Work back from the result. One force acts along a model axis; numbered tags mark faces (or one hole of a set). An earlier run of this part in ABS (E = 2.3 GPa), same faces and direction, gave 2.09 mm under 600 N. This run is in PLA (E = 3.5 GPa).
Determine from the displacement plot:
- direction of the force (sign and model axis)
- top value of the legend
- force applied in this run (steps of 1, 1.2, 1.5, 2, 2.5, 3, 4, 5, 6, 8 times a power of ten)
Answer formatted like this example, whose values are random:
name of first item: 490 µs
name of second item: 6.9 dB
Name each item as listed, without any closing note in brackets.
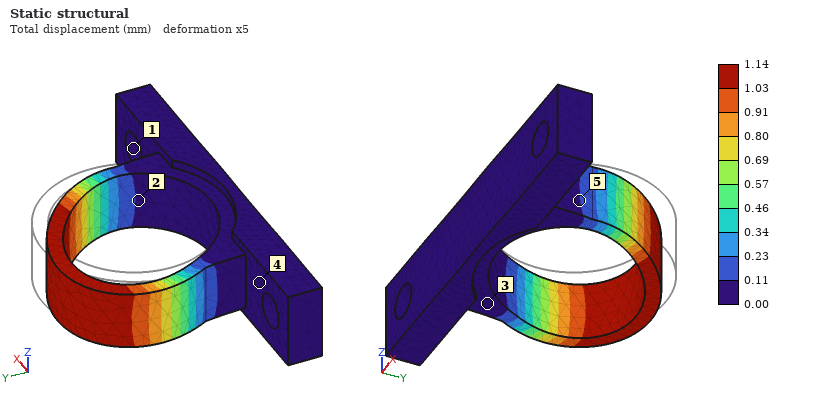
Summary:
direction of the force: -X
top value of the legend: 1.14 mm
force applied in this run: 500 N
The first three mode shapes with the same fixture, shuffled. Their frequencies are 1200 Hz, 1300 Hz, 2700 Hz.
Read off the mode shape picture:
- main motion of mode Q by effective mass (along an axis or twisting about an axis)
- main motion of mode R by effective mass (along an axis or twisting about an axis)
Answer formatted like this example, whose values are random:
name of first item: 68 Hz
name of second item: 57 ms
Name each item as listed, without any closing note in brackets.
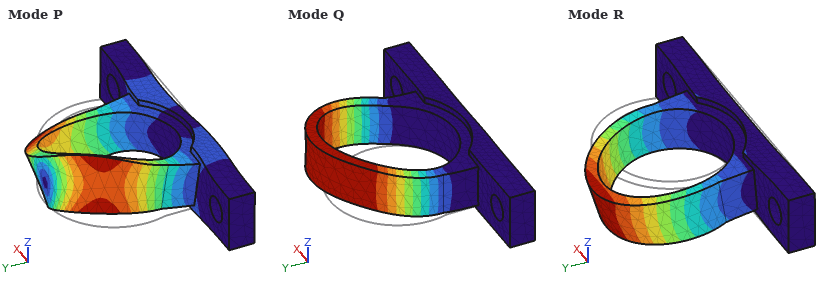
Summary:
main motion of mode Q by effective mass: along X
main motion of mode R by effective mass: along Z
